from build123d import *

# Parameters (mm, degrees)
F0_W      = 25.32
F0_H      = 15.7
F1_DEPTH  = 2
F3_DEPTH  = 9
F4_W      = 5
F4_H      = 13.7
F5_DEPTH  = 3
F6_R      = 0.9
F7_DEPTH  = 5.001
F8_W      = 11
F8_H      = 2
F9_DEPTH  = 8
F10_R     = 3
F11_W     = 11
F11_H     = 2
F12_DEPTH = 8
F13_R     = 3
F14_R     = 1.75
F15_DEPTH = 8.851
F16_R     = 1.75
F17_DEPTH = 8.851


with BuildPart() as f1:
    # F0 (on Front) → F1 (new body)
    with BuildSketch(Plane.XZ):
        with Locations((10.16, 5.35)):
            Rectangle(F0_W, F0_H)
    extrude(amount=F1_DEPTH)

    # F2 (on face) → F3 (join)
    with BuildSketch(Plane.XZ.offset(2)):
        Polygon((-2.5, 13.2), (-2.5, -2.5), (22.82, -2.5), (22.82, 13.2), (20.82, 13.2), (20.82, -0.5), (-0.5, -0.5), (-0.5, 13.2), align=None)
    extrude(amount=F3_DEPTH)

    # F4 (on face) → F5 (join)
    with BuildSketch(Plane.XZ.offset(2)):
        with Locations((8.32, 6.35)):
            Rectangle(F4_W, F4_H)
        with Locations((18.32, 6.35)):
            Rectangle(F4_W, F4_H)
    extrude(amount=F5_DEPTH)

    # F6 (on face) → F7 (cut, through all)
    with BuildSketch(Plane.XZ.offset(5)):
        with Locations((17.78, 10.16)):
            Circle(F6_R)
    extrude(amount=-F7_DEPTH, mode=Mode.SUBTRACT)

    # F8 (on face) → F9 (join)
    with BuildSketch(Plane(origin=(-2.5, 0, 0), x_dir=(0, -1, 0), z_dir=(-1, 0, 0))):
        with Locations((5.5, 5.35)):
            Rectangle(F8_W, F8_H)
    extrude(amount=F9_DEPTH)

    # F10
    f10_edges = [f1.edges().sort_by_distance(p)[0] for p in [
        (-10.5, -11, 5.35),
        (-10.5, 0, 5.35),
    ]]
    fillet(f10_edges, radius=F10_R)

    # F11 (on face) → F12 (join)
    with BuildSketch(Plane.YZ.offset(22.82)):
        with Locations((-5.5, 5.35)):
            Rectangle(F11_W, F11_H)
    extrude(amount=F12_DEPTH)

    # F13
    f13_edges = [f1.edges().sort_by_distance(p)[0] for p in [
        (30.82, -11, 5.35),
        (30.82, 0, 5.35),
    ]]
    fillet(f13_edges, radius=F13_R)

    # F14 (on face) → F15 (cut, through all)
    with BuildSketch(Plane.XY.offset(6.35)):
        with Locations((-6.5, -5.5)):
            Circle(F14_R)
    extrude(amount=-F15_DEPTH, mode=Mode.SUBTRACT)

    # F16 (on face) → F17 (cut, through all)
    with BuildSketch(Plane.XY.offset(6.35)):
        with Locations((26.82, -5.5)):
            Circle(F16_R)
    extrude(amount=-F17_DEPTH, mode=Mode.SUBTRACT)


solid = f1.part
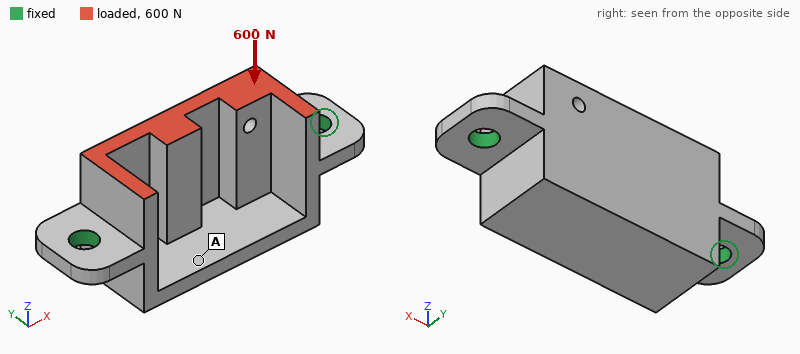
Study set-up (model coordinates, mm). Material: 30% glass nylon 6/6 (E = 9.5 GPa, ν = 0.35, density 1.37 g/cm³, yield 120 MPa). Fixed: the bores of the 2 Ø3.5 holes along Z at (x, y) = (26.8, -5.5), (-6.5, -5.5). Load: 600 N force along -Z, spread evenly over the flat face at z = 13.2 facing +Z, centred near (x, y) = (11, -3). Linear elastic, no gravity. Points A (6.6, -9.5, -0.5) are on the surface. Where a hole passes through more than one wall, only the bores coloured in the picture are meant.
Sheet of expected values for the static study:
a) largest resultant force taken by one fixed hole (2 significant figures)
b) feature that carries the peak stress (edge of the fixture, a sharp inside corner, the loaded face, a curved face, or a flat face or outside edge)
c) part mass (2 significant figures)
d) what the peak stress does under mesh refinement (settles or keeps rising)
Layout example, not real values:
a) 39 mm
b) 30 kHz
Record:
a) 320 N
b) edge of the fixture
c) 3.3 g
d) keeps rising
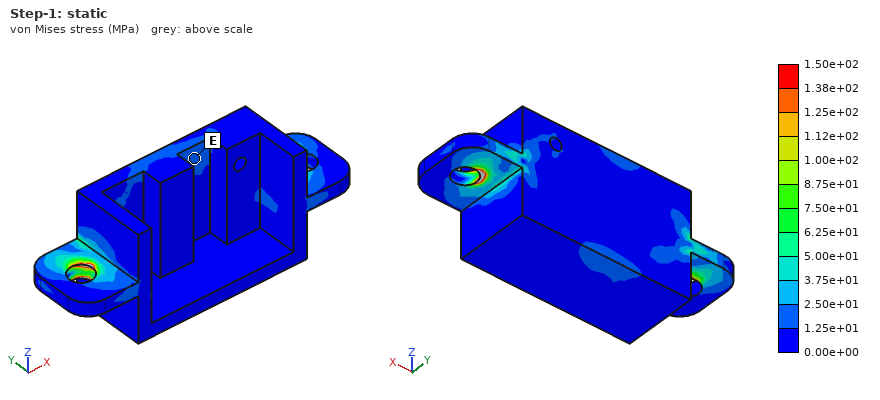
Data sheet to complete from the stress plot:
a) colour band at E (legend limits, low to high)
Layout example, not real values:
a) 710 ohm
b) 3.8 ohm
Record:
a) 1.25e+01 to 2.50e+01 MPa
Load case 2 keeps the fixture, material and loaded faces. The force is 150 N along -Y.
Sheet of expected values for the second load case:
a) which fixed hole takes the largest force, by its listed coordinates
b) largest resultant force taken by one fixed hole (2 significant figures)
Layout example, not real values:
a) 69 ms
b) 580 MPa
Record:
a) (26.8, -5.5)
b) 95 N
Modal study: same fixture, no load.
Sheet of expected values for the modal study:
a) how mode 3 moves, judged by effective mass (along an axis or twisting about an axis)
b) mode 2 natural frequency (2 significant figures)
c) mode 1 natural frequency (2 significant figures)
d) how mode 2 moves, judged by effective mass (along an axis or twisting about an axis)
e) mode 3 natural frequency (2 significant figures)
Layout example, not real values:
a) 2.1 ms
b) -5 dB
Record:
a) along Z
b) 8200 Hz
c) 4600 Hz
d) along Y
e) 8700 Hz
